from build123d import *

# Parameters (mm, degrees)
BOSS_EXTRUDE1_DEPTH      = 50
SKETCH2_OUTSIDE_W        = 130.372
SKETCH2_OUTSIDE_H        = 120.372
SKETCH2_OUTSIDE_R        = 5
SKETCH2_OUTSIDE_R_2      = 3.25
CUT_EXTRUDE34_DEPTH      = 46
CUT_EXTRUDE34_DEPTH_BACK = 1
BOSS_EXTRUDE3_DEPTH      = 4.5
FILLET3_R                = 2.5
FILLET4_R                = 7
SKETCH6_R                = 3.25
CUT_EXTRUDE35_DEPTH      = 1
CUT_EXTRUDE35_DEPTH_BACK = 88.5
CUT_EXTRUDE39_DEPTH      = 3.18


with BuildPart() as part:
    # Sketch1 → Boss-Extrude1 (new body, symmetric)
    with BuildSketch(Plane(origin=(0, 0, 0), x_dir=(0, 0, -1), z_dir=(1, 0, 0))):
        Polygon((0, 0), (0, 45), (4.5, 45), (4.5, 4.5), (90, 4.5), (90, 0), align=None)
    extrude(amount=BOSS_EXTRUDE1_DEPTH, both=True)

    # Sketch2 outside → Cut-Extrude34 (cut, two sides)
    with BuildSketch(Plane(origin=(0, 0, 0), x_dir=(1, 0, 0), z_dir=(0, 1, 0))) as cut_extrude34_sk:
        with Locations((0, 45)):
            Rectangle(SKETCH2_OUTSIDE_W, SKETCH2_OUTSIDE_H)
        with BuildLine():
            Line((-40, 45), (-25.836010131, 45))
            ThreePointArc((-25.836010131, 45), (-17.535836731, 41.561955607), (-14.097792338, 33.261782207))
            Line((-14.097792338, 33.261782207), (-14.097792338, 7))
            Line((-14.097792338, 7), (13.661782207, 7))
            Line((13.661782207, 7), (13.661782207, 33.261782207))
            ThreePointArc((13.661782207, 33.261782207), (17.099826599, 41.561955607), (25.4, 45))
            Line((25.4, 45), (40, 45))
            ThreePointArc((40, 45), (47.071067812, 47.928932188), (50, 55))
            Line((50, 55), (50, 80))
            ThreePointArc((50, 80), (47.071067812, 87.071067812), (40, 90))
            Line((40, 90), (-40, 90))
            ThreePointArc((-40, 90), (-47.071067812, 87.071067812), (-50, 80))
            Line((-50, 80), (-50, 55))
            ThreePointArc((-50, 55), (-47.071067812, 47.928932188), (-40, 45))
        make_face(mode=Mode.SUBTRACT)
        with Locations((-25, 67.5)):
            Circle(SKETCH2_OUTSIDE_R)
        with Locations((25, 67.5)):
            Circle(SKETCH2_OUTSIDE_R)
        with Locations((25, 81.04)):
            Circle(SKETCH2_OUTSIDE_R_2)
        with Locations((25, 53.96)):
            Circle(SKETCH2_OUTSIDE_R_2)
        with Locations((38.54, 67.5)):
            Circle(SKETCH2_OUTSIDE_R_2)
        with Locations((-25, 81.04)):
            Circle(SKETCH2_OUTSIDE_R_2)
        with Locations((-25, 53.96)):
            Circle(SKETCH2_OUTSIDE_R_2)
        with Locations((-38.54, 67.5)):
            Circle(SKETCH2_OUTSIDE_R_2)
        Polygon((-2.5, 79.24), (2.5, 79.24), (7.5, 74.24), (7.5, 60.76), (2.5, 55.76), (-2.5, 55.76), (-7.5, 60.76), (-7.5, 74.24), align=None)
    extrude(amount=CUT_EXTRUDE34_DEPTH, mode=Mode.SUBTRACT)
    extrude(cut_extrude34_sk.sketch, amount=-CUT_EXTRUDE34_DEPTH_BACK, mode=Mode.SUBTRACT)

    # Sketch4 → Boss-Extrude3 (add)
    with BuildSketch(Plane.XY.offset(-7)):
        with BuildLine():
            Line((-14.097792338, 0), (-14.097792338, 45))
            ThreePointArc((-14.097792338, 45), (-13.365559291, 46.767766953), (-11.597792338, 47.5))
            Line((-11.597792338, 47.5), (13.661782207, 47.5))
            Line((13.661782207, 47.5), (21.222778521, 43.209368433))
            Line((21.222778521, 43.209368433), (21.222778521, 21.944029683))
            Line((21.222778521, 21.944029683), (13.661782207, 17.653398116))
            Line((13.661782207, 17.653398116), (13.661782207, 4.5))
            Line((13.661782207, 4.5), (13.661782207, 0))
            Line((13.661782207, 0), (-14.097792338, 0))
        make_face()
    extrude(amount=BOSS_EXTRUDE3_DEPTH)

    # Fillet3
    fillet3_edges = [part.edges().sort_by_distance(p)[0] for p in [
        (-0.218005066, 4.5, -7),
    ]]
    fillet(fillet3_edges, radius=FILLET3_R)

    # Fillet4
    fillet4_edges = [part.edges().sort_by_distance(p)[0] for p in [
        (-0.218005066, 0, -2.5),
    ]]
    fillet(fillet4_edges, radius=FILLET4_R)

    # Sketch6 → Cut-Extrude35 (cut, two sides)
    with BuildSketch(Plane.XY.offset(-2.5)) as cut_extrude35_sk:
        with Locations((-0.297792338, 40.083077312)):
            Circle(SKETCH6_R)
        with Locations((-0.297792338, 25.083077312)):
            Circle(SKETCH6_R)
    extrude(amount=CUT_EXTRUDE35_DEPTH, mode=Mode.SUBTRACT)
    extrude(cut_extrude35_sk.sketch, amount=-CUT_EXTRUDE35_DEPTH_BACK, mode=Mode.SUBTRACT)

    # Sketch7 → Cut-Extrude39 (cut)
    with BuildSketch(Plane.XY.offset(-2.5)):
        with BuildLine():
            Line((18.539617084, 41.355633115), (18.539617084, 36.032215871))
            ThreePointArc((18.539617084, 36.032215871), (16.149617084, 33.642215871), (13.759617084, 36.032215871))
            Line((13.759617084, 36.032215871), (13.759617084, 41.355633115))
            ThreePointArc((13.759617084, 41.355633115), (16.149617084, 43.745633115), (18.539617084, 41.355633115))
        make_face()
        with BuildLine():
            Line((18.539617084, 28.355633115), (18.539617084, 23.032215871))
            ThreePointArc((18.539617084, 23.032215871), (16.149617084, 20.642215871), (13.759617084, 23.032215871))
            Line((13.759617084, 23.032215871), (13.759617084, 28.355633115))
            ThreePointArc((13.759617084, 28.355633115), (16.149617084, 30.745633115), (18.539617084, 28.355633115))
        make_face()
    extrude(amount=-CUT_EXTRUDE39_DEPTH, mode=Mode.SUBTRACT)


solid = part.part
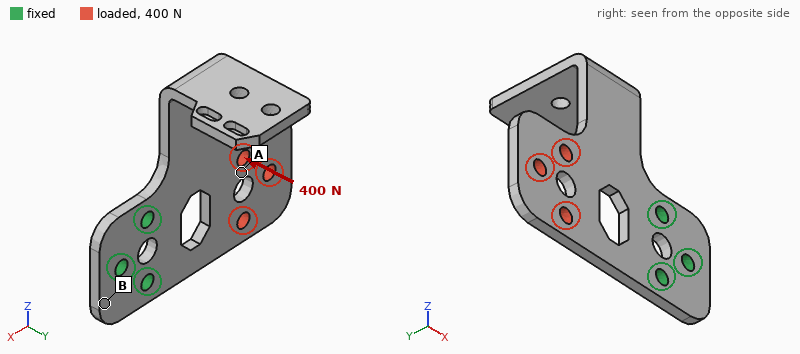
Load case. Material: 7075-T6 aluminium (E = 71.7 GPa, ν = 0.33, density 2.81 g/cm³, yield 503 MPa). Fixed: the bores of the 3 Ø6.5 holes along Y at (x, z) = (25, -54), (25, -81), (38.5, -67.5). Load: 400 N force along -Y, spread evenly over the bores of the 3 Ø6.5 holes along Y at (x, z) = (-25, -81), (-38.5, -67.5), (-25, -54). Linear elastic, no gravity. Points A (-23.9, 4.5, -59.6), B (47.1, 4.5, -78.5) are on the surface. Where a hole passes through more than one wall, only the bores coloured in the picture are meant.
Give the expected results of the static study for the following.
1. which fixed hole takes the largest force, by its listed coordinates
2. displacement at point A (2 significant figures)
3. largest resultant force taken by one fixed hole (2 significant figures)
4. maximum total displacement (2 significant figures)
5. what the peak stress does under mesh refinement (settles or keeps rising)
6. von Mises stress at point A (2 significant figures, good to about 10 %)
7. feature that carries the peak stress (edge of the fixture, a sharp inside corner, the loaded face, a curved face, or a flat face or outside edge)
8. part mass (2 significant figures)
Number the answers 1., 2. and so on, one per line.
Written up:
1. (25, -54)
2. 0.80 mm
3. 280 N
4. 1.5 mm
5. keeps rising
6. 32 MPa
7. edge of the fixture
8. 78 g
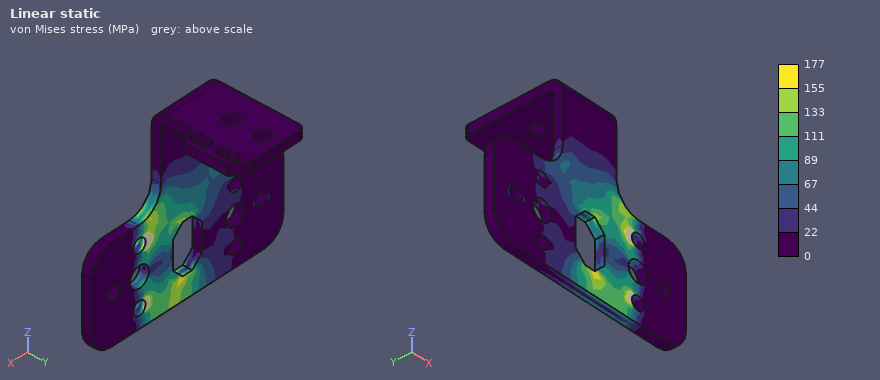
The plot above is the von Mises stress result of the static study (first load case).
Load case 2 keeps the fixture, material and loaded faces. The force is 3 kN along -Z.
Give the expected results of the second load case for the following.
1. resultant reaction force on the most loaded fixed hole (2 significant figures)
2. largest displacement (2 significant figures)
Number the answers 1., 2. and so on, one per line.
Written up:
1. 5.0 kN
2. 0.20 mm
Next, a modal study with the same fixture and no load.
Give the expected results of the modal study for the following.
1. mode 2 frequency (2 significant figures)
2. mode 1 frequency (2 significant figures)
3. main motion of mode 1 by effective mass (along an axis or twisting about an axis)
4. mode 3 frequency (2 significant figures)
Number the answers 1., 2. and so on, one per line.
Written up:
1. 590 Hz
2. 470 Hz
3. along Y
4. 1000 Hz
